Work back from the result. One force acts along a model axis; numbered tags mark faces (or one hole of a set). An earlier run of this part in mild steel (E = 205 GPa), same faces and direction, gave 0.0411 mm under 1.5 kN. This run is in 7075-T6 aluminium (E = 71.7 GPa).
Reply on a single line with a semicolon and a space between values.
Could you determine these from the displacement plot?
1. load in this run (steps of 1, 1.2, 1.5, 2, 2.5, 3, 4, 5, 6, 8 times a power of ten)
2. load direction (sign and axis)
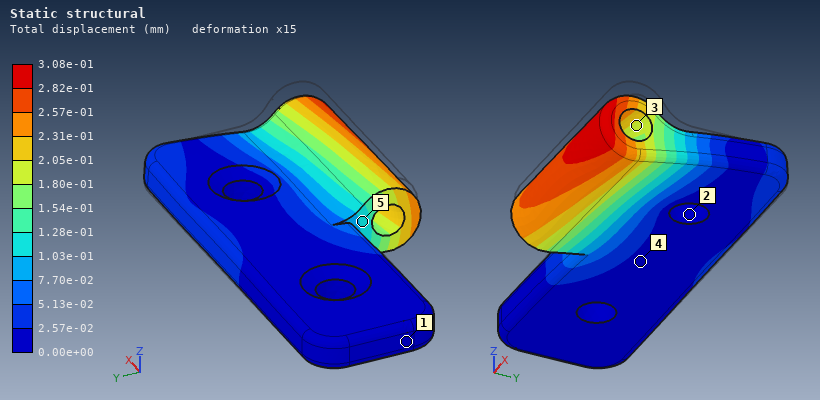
4 kN; -Z
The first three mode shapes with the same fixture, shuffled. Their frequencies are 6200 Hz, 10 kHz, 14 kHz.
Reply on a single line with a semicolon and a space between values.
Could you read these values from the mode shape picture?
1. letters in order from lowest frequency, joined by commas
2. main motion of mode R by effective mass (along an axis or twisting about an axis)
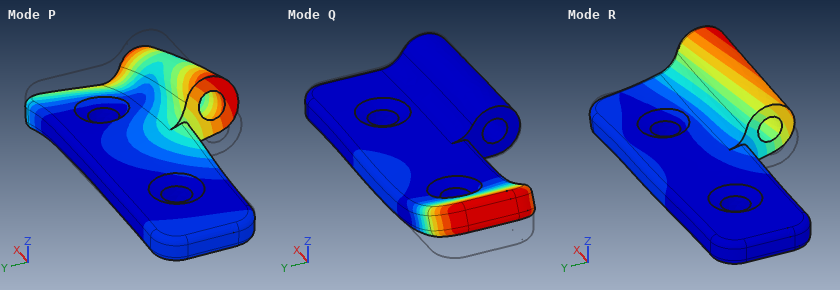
R, P, Q; along Z
